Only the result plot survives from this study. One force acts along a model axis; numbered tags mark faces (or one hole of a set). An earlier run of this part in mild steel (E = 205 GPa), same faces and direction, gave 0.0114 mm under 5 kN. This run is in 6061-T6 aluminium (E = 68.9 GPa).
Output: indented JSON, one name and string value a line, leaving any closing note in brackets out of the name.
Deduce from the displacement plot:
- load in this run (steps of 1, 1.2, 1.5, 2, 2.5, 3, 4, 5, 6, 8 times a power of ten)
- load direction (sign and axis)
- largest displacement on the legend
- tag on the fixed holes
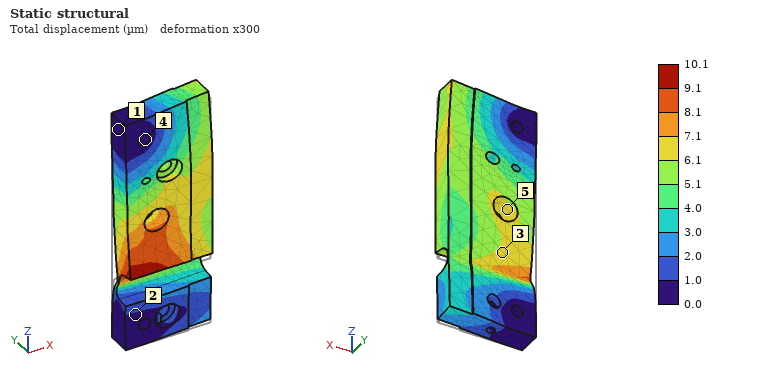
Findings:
{
  "load in this run": "1.5 kN",
  "load direction": "+Z",
  "largest displacement on the legend": "10.1 µm",
  "tag on the fixed holes": "4"
}
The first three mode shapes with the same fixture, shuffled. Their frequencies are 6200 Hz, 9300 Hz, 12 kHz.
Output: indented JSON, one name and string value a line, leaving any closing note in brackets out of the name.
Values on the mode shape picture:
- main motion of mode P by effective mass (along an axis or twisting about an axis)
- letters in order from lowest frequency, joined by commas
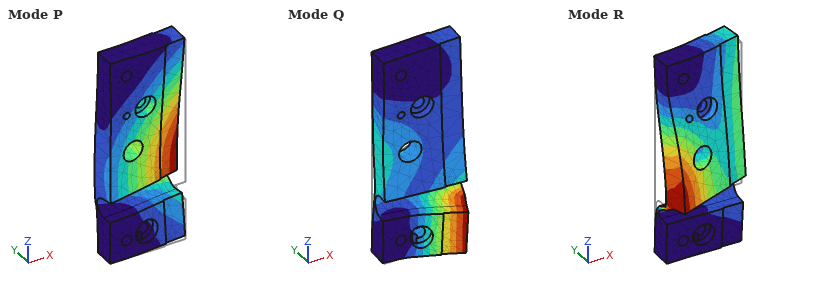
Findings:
{
  "main motion of mode P by effective mass": "along Y",
  "letters in order from lowest frequency, joined by commas": "P, R, Q"
}
